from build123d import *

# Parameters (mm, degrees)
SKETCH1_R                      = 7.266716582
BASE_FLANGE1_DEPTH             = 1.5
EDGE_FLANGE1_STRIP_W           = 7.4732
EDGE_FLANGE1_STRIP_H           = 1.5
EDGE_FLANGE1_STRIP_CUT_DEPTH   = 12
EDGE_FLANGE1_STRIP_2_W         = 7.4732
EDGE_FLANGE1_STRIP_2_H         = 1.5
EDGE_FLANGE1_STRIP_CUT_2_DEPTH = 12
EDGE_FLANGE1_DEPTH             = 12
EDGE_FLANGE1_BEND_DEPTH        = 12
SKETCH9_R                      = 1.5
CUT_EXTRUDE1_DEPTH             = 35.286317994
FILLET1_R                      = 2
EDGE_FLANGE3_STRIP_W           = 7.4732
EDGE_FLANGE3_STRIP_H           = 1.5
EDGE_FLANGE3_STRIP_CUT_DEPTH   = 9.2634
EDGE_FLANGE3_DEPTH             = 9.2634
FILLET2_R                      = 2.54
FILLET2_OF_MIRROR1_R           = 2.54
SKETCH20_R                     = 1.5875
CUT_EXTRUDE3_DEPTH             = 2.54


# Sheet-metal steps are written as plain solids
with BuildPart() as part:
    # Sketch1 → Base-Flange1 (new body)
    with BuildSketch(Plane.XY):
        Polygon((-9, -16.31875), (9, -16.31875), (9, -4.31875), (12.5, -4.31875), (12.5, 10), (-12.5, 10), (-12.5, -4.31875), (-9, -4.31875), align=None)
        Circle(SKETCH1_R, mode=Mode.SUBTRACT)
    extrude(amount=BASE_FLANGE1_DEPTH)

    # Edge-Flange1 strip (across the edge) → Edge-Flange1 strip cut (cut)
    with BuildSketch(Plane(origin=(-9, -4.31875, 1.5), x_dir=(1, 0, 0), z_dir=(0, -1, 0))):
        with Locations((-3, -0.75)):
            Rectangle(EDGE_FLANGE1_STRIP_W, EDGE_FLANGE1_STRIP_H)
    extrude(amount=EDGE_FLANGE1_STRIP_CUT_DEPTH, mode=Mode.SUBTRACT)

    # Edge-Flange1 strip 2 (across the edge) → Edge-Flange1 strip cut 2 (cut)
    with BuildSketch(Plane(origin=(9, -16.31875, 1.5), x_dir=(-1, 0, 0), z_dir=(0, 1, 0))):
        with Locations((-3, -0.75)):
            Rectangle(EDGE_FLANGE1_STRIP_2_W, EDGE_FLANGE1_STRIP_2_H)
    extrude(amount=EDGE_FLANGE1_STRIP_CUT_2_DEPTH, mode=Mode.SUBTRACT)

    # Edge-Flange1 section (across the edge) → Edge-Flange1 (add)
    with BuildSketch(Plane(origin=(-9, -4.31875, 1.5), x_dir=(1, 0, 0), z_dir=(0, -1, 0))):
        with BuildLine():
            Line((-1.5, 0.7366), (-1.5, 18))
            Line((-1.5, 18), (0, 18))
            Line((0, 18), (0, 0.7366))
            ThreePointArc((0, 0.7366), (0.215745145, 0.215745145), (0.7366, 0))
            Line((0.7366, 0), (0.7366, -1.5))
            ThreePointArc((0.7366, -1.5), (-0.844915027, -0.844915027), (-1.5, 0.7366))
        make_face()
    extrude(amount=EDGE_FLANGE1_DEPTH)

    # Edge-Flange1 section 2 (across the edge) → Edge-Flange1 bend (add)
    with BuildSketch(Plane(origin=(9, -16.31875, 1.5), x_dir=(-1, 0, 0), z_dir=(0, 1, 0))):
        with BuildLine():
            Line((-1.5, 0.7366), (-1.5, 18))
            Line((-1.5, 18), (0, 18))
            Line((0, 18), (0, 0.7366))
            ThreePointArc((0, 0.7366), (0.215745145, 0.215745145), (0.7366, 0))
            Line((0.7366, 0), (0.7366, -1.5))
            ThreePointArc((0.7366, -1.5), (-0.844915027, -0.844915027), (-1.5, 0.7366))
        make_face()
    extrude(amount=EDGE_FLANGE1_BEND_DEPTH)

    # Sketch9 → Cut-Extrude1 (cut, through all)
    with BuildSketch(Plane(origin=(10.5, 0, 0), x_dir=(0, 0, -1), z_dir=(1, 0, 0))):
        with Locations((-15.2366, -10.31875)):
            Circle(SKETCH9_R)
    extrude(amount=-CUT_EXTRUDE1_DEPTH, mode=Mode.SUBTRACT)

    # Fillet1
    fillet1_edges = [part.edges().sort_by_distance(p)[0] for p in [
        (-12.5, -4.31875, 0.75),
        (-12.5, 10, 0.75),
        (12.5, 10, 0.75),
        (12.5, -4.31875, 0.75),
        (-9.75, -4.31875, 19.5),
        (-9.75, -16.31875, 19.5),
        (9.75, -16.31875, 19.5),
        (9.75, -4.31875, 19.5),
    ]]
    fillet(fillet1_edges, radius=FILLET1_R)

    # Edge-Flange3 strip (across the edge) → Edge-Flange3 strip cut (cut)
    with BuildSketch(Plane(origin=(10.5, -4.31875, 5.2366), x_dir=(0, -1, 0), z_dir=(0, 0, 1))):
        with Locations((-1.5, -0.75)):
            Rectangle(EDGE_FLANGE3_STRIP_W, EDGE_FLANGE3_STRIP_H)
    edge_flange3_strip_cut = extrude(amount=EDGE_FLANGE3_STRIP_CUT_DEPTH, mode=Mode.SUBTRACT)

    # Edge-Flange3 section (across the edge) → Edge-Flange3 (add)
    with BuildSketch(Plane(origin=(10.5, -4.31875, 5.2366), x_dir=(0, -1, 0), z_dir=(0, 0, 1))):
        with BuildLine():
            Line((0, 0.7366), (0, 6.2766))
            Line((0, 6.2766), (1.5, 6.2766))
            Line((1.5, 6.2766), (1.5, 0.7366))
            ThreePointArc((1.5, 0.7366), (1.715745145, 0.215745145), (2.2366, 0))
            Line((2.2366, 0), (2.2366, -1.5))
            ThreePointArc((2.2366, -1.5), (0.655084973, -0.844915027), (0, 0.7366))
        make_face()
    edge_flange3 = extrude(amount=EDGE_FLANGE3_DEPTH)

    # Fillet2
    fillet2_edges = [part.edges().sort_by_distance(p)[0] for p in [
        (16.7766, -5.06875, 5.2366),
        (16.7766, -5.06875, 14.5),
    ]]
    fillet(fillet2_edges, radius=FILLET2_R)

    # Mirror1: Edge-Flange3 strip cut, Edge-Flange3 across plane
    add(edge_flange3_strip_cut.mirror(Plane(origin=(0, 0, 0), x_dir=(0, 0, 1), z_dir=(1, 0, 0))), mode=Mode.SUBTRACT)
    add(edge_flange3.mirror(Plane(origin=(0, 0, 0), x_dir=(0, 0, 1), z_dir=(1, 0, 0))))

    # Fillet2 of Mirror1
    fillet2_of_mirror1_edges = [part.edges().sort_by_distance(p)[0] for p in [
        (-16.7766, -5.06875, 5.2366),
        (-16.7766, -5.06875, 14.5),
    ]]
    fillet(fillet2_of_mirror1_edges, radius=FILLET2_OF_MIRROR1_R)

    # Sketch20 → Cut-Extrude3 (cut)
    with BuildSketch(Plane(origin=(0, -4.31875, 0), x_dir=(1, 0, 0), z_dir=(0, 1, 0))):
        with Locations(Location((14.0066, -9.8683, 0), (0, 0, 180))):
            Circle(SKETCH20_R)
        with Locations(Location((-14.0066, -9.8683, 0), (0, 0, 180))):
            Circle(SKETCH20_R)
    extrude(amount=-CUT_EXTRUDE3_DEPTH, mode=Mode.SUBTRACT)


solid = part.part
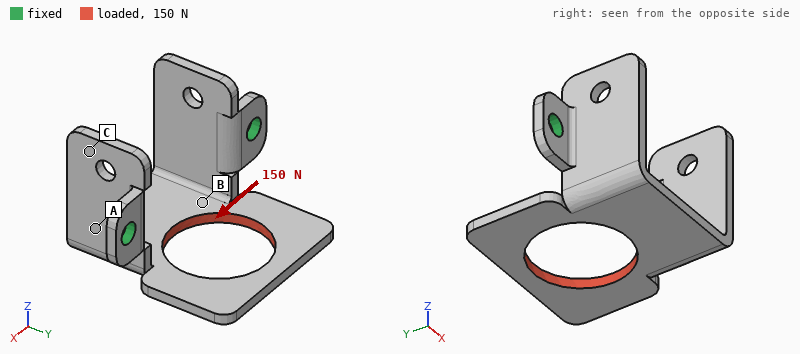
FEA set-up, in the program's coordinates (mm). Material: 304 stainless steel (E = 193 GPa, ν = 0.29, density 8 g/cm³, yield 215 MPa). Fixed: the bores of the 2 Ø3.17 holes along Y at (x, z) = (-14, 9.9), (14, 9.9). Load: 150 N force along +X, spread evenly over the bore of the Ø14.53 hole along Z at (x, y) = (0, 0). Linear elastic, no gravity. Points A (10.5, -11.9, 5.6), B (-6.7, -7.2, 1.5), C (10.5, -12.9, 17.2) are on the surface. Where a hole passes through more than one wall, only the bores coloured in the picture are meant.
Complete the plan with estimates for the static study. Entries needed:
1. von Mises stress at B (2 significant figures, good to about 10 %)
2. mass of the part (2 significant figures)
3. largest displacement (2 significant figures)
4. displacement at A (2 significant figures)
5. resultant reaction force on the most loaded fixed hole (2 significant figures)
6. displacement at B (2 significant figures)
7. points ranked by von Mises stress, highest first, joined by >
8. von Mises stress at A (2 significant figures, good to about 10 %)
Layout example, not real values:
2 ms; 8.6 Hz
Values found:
43 MPa; 11 g; 36 µm; 7.4 µm; 85 N; 12 µm; B > A > C; 24 MPa
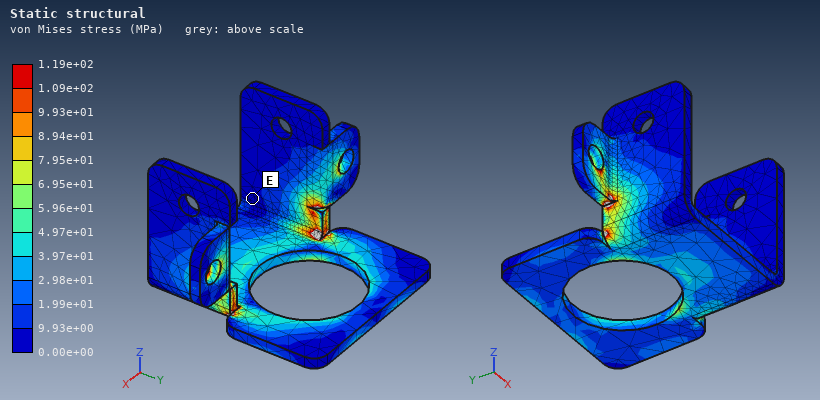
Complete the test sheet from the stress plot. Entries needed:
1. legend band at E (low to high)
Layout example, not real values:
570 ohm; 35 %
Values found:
0.00e+00 to 9.93e+00 MPa
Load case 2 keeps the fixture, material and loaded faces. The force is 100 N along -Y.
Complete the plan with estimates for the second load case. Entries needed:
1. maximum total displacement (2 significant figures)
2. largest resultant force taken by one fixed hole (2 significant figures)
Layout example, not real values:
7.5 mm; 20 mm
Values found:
25 µm; 52 N
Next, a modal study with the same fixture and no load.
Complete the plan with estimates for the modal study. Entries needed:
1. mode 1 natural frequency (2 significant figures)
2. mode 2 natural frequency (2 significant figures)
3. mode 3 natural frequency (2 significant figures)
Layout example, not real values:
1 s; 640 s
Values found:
2700 Hz; 4700 Hz; 5000 Hz
